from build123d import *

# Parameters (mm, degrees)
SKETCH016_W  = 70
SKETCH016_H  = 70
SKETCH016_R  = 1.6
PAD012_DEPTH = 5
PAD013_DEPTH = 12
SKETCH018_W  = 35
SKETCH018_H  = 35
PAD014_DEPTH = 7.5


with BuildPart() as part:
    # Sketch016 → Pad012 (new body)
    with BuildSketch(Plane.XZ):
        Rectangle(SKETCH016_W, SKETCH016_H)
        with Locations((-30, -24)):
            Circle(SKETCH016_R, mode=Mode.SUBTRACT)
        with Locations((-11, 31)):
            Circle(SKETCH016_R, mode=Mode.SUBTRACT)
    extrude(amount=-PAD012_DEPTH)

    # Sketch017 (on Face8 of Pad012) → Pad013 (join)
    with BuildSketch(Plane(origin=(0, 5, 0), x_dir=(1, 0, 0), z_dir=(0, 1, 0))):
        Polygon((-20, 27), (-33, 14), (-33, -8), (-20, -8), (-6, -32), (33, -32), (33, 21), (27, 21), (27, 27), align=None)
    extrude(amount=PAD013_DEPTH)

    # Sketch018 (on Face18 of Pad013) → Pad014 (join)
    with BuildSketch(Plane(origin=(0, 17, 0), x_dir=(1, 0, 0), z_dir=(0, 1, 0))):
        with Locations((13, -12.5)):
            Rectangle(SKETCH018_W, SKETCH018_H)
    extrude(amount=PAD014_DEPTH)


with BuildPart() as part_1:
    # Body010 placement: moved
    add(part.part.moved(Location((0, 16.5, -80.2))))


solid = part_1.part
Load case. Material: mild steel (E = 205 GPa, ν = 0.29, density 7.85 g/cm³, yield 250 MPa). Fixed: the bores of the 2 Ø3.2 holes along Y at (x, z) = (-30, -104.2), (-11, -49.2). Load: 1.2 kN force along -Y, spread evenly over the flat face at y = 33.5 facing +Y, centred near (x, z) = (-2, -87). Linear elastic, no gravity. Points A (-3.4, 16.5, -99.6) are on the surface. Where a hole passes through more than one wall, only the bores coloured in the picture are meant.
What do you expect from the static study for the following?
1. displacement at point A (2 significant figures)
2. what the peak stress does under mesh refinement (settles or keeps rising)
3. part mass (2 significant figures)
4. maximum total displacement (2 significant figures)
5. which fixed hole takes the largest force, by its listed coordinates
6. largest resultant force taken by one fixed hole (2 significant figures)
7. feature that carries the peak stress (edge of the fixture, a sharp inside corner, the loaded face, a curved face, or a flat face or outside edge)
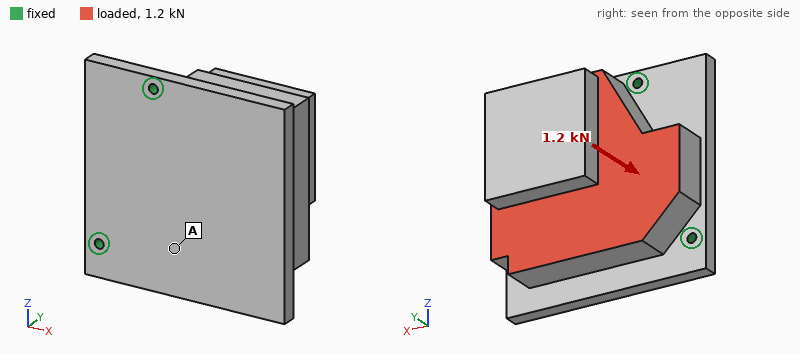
0.039 mm
keeps rising
570 g
0.11 mm
(-30, -104.2)
700 N
edge of the fixture
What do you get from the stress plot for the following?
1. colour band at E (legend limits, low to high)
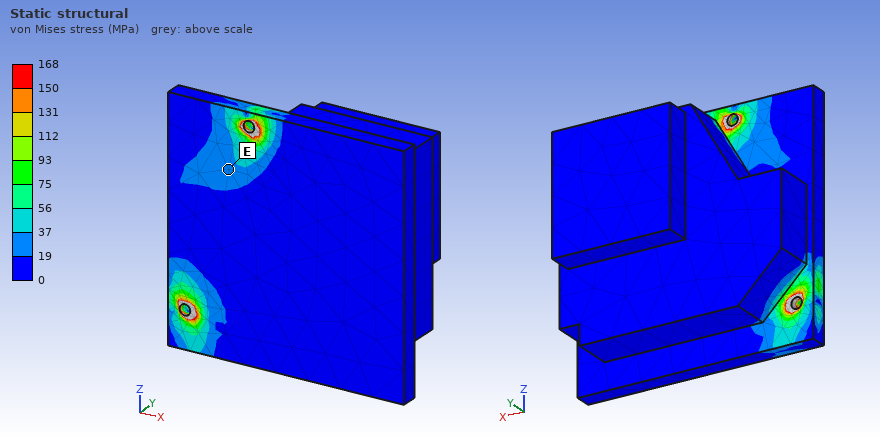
19 to 37 MPa
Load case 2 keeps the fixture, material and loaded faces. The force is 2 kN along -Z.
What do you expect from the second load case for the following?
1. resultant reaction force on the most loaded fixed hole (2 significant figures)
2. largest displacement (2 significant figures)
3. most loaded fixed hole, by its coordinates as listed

1.4 kN
46 µm
(-11, -49.2)
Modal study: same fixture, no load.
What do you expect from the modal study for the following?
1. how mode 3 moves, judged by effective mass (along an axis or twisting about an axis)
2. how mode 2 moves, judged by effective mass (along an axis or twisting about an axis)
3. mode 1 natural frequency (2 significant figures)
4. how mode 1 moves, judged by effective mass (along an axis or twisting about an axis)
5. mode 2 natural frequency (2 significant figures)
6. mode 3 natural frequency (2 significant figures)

along Z
along Z
840 Hz
along Y
6100 Hz
6400 Hz
